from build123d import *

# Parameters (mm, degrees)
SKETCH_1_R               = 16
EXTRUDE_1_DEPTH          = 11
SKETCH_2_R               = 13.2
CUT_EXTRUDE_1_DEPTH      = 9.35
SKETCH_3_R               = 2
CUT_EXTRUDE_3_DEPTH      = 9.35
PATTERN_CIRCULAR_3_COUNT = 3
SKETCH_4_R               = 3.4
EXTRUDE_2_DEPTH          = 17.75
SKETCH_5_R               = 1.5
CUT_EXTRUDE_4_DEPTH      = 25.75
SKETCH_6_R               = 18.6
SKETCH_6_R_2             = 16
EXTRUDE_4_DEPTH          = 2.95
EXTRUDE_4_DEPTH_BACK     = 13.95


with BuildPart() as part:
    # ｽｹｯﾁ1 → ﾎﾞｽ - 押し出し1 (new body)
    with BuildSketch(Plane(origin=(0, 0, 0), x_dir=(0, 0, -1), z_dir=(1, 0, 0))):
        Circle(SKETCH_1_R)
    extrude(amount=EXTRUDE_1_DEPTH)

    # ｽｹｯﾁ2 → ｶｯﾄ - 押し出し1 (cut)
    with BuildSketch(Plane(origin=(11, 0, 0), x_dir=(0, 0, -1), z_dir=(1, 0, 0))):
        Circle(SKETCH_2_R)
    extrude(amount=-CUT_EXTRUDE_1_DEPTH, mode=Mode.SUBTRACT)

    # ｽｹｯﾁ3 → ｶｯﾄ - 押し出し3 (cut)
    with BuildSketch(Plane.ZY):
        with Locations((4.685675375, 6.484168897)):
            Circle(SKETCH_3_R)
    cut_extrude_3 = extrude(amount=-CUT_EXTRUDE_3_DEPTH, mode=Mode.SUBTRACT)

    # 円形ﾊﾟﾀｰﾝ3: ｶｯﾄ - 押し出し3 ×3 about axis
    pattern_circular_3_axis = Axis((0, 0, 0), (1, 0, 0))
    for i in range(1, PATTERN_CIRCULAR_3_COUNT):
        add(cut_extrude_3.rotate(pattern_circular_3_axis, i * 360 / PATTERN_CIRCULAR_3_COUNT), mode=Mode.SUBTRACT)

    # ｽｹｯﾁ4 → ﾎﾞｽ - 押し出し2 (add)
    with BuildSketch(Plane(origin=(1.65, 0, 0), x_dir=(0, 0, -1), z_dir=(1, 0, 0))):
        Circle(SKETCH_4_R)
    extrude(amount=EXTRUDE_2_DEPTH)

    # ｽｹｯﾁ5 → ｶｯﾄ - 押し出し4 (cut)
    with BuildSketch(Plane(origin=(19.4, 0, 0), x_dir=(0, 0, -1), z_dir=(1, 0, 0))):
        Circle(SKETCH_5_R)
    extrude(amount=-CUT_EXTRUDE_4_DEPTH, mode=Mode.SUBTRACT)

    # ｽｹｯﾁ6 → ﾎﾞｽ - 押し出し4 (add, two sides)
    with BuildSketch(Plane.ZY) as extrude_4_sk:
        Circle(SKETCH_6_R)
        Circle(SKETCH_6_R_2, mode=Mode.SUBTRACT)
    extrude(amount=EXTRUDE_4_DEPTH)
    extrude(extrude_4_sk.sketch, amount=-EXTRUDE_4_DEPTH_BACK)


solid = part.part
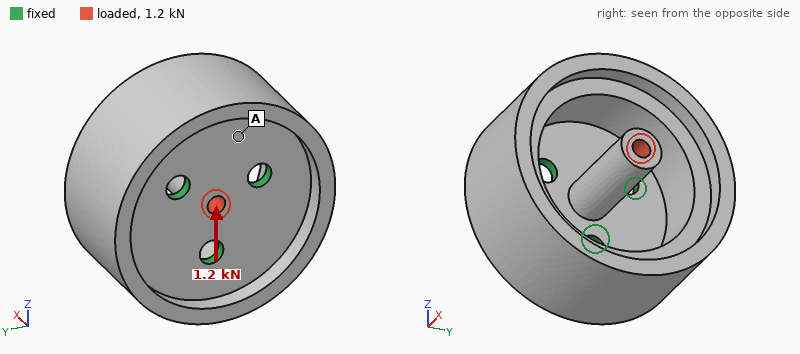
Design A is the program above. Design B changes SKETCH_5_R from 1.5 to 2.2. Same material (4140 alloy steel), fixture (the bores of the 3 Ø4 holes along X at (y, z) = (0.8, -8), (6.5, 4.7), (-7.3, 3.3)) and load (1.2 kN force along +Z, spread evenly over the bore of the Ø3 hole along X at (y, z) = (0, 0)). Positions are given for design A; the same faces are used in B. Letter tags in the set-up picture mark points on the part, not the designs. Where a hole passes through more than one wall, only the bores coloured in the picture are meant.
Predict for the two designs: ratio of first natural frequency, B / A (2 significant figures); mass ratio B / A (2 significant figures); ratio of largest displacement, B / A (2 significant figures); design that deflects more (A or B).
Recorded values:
1.00
0.98
1.2
B
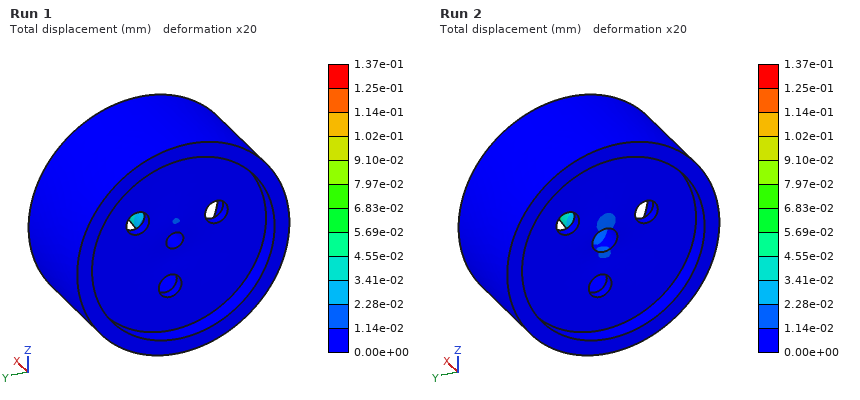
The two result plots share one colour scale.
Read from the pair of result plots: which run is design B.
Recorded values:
Run 2
